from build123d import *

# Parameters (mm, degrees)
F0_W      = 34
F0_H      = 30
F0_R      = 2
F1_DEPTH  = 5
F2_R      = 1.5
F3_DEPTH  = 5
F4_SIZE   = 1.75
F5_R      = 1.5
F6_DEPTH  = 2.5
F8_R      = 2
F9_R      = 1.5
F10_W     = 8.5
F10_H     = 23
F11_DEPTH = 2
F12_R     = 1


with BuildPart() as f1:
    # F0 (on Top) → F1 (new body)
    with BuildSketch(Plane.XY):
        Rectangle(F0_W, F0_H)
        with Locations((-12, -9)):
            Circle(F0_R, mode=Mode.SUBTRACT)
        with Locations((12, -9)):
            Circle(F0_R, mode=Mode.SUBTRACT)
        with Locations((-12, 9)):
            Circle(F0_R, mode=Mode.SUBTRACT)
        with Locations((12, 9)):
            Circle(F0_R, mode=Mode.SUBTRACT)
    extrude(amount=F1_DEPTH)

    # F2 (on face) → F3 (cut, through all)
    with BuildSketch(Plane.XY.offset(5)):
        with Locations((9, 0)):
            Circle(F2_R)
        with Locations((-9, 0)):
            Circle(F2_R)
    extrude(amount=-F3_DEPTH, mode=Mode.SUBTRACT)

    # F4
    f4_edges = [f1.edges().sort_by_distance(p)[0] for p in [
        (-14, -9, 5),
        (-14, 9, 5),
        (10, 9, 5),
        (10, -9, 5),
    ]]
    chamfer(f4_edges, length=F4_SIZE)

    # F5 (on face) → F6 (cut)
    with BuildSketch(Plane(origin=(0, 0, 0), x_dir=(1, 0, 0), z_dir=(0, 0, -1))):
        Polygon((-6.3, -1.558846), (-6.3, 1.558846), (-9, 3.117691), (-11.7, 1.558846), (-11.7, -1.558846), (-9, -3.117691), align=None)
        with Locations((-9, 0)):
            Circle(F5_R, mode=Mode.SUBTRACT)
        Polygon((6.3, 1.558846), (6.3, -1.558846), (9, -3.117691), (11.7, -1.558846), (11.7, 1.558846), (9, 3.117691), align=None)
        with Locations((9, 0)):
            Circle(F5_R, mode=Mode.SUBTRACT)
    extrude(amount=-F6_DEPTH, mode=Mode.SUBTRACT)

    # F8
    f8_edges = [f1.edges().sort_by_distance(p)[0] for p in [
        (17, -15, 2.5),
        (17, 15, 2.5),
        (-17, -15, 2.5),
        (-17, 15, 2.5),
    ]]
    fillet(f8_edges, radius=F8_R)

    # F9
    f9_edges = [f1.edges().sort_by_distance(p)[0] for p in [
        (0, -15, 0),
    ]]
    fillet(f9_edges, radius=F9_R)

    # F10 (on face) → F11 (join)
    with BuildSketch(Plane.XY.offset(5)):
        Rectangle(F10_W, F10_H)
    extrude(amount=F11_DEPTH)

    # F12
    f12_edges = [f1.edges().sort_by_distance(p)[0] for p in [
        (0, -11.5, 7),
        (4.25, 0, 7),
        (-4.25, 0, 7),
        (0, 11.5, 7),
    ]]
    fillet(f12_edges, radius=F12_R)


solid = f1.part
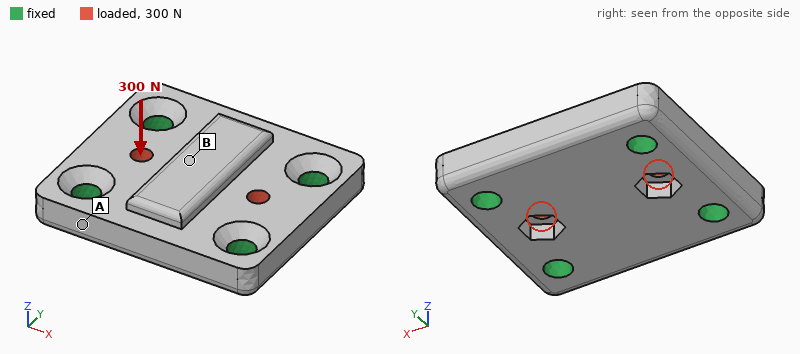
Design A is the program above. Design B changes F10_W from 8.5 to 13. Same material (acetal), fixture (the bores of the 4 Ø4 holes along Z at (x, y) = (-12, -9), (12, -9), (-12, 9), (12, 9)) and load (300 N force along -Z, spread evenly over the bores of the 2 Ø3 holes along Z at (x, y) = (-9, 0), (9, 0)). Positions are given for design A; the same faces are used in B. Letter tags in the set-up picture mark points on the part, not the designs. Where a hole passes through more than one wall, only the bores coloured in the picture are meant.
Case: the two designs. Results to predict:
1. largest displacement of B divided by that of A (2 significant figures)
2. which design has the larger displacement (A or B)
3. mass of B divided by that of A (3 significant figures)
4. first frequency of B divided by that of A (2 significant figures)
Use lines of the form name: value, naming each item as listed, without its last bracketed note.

largest displacement of B divided by that of A: 0.90
which design has the larger displacement: A
mass of B divided by that of A: 1.04
first frequency of B divided by that of A: 1.0
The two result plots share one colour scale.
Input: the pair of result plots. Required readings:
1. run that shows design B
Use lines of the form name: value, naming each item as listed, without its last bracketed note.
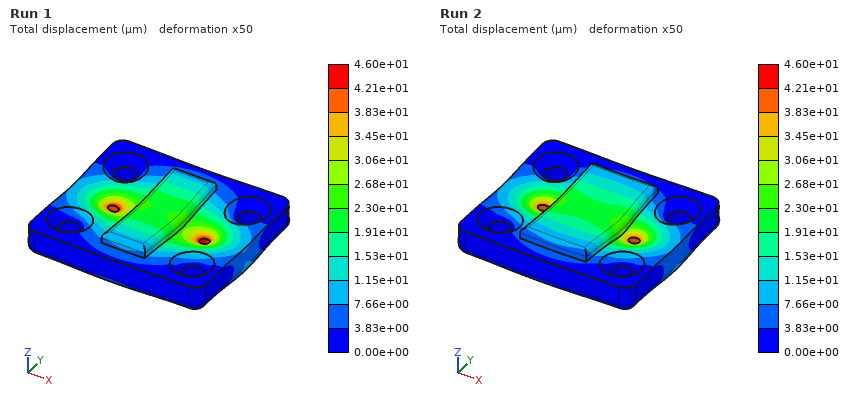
run that shows design B: Run 2
